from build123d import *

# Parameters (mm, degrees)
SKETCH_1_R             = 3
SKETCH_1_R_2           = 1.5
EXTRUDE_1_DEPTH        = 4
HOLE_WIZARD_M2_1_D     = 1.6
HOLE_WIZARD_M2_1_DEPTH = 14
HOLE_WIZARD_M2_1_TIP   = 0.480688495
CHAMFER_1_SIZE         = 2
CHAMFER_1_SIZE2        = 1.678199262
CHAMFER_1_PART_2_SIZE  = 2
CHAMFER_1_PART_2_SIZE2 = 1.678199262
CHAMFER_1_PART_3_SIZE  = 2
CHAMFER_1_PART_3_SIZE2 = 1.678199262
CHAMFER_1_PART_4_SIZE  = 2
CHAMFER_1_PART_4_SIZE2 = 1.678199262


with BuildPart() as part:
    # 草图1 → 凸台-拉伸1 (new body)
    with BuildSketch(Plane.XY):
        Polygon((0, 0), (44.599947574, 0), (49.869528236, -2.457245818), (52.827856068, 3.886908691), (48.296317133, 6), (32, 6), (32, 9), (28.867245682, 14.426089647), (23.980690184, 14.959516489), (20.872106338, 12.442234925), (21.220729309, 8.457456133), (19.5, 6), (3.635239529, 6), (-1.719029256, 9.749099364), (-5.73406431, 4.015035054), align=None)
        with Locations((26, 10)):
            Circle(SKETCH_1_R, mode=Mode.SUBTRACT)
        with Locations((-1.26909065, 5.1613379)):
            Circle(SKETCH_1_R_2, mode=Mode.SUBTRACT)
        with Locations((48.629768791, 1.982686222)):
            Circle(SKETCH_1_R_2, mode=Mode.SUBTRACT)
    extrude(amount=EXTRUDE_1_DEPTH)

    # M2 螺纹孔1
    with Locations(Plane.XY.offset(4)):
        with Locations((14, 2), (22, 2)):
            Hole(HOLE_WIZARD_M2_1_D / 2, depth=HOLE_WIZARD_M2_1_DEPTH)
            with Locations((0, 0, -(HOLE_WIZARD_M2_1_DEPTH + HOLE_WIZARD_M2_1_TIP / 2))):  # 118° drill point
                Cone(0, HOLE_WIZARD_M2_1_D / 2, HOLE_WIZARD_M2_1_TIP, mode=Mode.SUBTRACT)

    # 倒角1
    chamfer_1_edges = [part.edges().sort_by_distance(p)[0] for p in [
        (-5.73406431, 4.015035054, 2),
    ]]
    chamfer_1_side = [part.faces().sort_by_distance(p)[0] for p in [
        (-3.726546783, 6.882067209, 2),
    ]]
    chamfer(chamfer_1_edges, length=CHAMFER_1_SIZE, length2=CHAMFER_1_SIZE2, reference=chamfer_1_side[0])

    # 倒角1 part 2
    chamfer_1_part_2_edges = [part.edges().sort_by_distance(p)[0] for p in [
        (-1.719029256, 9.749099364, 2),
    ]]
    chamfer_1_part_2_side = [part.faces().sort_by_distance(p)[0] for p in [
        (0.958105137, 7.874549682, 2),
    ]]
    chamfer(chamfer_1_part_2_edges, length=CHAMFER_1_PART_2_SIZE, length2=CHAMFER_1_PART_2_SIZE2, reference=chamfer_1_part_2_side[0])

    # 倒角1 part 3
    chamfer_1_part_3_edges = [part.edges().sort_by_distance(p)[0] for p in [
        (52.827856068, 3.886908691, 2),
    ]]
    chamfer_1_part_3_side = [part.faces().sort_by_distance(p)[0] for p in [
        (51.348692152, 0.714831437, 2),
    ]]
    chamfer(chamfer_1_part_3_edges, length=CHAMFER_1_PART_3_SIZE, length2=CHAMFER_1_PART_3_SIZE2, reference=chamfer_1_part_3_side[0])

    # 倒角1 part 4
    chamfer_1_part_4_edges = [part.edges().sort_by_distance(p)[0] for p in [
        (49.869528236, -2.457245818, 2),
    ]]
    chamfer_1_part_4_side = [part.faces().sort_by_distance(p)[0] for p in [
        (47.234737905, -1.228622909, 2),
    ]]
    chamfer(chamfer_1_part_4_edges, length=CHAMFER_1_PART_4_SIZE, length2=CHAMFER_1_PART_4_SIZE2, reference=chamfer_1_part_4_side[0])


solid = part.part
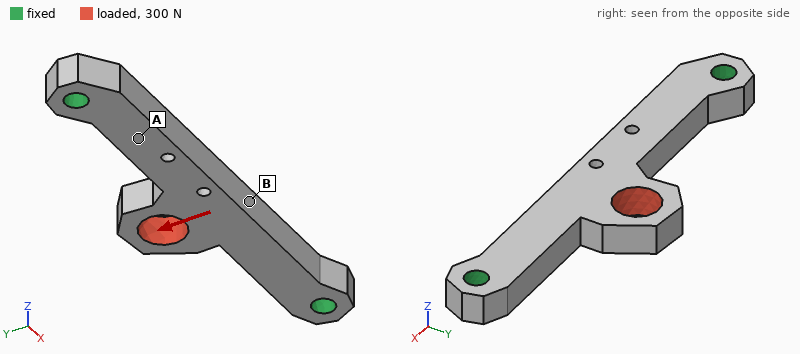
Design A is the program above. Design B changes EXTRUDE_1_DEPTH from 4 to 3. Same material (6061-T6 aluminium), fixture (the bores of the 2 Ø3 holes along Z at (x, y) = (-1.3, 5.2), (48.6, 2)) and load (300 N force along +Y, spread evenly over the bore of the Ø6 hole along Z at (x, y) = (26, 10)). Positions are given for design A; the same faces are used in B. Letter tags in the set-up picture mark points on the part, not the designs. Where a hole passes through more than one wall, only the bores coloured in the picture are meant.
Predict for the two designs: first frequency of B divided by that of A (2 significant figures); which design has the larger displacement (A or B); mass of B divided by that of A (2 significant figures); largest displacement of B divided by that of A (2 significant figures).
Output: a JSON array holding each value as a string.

["0.78", "B", "0.75", "1.3"]
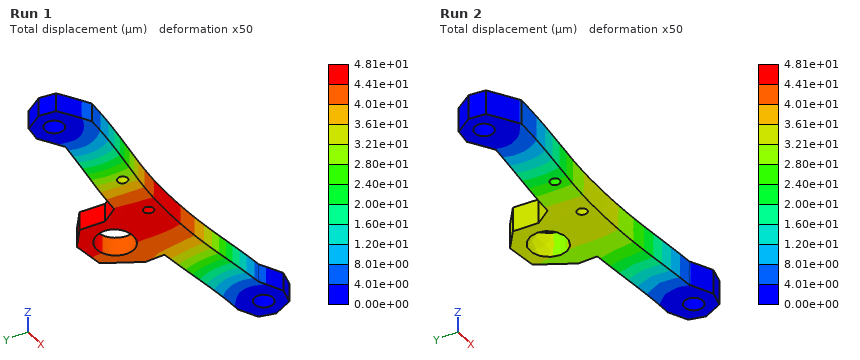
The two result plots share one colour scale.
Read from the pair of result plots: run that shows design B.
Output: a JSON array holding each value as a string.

["Run 1"]
